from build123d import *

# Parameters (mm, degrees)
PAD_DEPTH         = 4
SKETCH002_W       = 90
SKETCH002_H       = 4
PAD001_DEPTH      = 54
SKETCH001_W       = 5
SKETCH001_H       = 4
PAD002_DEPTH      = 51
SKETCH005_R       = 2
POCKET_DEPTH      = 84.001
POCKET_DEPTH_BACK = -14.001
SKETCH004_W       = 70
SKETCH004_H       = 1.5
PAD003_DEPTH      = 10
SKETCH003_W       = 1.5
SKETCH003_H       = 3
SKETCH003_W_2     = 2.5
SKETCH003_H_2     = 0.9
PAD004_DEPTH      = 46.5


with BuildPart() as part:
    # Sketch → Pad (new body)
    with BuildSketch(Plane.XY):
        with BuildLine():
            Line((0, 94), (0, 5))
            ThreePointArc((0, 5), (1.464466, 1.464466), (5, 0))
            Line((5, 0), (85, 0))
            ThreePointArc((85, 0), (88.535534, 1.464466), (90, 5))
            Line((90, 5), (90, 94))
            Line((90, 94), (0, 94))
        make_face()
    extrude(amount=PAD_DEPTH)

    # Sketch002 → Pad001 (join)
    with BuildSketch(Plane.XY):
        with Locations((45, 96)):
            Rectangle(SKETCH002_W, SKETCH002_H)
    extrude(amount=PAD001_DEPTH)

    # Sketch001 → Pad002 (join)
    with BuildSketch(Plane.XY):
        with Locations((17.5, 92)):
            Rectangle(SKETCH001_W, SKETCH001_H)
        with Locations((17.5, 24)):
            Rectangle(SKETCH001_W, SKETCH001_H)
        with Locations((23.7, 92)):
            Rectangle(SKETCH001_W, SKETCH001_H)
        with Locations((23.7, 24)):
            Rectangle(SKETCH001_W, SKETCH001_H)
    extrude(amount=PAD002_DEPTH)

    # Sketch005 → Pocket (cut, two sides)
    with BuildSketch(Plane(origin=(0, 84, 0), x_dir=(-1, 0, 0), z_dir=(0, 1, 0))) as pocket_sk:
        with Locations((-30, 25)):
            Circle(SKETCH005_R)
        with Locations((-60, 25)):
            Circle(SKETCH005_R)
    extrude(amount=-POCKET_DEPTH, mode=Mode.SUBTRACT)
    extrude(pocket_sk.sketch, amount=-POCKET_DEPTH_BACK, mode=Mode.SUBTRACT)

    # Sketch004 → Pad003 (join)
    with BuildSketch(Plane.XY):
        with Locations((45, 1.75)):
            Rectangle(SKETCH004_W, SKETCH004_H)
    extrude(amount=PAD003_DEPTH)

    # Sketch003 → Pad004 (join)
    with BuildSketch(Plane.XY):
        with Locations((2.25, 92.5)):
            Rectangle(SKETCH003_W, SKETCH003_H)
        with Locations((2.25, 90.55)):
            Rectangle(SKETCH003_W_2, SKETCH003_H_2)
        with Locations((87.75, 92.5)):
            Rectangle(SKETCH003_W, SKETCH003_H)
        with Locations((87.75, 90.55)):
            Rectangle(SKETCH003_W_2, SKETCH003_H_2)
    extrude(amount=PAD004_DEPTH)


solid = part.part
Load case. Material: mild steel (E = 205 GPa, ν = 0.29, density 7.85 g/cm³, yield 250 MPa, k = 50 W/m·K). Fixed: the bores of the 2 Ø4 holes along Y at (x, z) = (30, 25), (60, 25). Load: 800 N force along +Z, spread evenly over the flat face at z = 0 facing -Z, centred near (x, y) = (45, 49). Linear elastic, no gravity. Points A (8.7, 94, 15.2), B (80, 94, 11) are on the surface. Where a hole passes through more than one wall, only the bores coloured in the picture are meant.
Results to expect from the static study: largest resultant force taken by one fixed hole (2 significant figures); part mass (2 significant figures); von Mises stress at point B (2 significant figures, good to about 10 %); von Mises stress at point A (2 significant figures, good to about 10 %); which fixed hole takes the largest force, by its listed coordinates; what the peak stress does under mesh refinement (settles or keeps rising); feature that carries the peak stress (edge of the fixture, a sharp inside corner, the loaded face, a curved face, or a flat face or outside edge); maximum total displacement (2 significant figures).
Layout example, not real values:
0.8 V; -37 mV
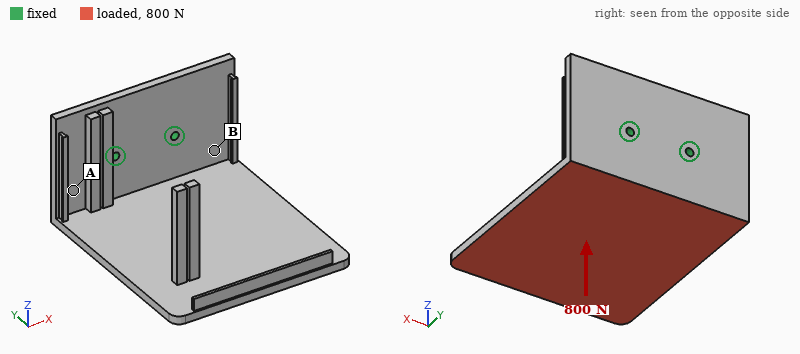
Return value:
450 N; 460 g; 71 MPa; 25 MPa; (60, 25); keeps rising; edge of the fixture; 1.4 mm
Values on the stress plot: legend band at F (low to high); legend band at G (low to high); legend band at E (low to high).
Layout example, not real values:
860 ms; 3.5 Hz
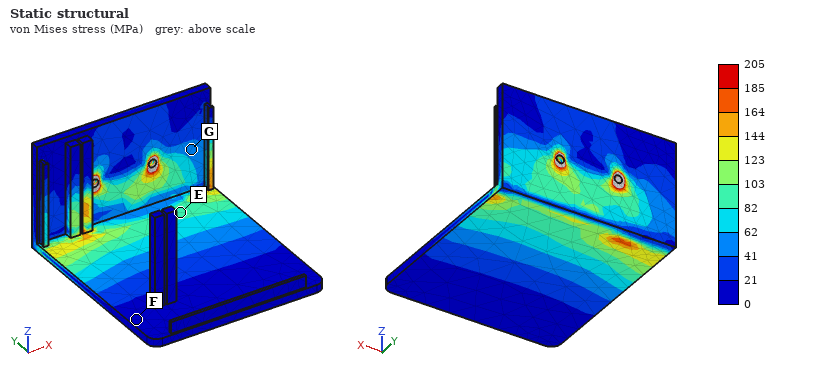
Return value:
0 to 21 MPa; 41 to 62 MPa; 82 to 103 MPa
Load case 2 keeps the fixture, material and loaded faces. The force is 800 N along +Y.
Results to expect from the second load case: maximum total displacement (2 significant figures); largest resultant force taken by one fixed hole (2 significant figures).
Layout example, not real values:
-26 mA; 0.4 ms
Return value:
0.27 mm; 420 N
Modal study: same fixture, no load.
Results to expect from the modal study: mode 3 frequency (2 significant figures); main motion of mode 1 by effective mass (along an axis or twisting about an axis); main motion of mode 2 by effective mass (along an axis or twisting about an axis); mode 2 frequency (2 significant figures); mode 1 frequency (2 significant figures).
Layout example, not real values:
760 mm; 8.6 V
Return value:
880 Hz; along Z; along X; 570 Hz; 260 Hz
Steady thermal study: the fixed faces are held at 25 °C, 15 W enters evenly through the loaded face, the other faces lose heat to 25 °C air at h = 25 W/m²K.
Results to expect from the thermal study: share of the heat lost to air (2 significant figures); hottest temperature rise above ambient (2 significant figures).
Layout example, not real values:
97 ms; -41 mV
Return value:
56 %; 28 K
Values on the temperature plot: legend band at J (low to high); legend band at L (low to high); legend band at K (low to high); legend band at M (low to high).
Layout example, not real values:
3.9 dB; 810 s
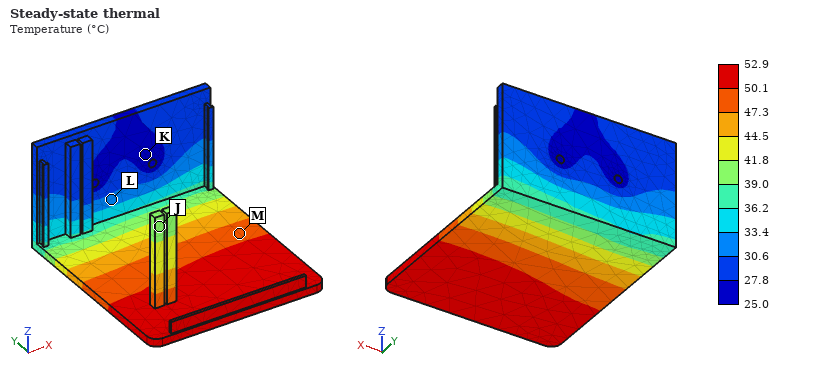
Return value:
39.0 to 41.8 °C; 30.6 to 33.4 °C; 25.0 to 27.8 °C; 47.3 to 50.1 °C
